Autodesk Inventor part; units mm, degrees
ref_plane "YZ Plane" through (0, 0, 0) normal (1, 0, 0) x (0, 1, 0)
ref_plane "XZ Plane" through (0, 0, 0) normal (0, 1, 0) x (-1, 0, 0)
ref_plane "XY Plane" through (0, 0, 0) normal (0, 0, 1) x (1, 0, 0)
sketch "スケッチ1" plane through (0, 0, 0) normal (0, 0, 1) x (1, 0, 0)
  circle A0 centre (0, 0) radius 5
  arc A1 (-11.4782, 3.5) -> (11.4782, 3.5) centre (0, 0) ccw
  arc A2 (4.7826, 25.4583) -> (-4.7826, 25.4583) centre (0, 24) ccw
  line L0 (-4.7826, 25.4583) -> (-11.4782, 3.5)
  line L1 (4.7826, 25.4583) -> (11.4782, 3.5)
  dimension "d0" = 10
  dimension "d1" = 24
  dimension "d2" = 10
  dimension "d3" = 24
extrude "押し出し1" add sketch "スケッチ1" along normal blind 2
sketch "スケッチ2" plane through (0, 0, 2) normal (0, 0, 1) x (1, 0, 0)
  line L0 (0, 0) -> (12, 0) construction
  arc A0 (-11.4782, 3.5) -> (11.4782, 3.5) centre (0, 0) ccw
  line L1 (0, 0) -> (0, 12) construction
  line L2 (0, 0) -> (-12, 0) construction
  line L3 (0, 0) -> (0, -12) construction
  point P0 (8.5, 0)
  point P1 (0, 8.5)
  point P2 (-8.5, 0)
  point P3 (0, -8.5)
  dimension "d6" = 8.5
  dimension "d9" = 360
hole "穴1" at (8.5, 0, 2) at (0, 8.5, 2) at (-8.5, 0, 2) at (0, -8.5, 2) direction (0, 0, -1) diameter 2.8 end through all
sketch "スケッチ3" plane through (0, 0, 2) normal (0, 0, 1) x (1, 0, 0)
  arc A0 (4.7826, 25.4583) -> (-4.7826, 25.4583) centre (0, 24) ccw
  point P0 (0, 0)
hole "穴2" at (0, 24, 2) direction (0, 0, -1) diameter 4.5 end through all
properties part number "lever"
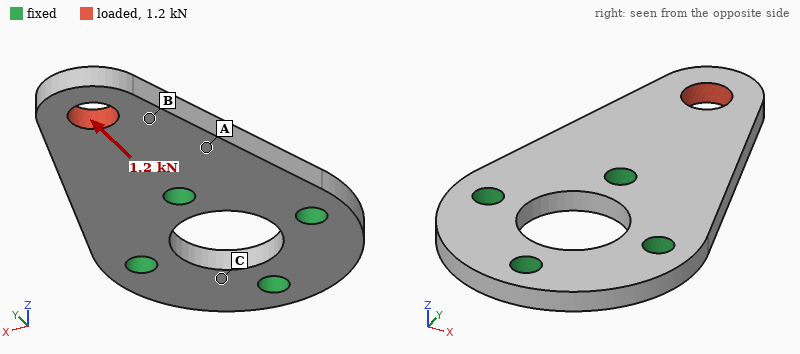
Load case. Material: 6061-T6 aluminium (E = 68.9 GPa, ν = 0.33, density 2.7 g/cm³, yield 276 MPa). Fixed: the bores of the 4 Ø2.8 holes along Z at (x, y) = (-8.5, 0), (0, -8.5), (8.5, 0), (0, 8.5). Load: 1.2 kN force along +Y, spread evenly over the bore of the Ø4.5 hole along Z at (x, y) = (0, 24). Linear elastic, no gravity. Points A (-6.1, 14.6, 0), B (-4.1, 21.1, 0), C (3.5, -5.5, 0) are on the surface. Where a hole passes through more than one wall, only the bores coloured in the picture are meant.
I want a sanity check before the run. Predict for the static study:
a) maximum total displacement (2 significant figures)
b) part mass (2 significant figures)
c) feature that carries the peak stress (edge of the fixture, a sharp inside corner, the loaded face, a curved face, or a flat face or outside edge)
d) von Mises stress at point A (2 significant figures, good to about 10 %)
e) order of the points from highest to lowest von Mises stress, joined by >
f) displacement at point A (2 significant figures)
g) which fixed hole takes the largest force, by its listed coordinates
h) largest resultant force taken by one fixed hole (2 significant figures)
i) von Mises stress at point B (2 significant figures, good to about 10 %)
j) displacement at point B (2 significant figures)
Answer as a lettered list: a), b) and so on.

a) 17 µm
b) 3.1 g
c) the loaded face
d) 31 MPa
e) B > A > C
f) 4.5 µm
g) (0, 8.5)
h) 760 N
i) 56 MPa
j) 8.6 µm
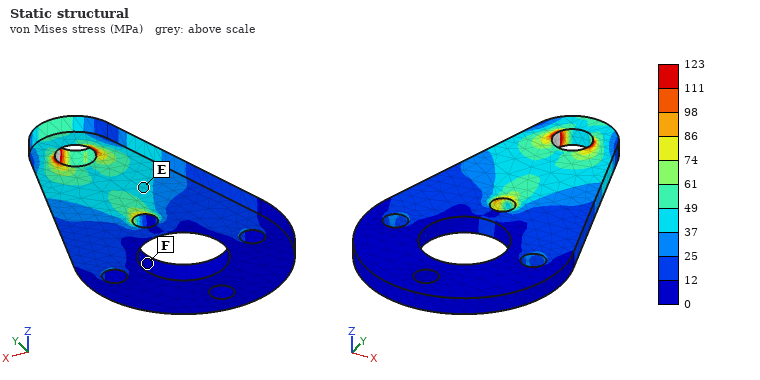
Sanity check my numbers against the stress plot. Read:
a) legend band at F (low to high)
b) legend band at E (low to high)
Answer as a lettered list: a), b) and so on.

a) 0 to 12 MPa
b) 37 to 49 MPa
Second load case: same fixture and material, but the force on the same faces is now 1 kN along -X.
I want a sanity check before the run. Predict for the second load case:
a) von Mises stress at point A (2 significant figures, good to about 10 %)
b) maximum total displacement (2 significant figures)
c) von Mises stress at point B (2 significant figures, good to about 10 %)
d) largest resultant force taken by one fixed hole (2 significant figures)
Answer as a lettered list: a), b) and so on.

a) 94 MPa
b) 86 µm
c) 58 MPa
d) 920 N
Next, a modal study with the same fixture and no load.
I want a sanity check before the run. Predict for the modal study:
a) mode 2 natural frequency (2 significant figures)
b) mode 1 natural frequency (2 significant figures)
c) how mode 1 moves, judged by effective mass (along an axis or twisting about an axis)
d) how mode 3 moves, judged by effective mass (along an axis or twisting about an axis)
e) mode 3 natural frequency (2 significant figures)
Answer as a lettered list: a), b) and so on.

a) 15 kHz
b) 5800 Hz
c) along Z
d) along Z
e) 23 kHz
